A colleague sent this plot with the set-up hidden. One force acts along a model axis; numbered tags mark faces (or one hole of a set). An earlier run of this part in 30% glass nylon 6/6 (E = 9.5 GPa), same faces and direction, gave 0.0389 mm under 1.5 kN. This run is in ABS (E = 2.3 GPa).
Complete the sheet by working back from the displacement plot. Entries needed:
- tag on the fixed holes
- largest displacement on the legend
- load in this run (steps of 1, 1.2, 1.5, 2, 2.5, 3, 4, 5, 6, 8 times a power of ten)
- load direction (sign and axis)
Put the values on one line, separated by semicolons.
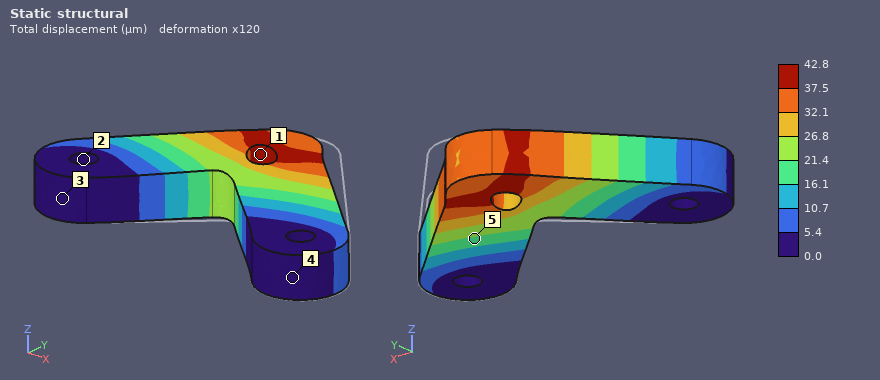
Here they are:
2; 42.8 µm; 400 N; -X
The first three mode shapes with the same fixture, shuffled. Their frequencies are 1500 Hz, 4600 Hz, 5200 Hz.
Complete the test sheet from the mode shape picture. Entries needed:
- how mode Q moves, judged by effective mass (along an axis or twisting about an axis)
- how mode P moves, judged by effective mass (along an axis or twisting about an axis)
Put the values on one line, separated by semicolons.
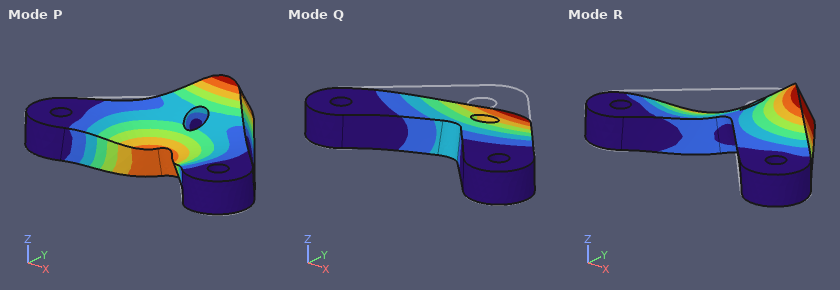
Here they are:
along Z; along Z
